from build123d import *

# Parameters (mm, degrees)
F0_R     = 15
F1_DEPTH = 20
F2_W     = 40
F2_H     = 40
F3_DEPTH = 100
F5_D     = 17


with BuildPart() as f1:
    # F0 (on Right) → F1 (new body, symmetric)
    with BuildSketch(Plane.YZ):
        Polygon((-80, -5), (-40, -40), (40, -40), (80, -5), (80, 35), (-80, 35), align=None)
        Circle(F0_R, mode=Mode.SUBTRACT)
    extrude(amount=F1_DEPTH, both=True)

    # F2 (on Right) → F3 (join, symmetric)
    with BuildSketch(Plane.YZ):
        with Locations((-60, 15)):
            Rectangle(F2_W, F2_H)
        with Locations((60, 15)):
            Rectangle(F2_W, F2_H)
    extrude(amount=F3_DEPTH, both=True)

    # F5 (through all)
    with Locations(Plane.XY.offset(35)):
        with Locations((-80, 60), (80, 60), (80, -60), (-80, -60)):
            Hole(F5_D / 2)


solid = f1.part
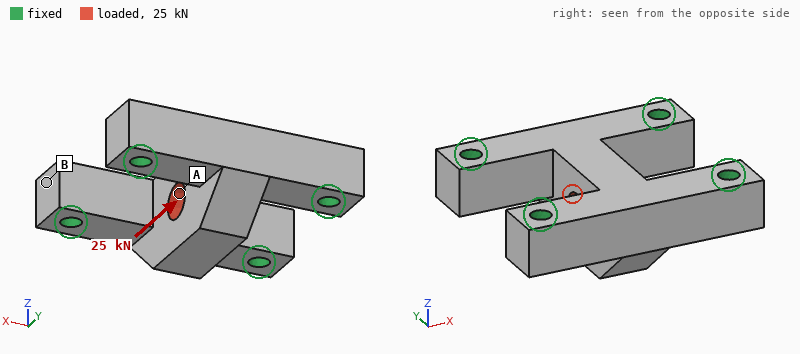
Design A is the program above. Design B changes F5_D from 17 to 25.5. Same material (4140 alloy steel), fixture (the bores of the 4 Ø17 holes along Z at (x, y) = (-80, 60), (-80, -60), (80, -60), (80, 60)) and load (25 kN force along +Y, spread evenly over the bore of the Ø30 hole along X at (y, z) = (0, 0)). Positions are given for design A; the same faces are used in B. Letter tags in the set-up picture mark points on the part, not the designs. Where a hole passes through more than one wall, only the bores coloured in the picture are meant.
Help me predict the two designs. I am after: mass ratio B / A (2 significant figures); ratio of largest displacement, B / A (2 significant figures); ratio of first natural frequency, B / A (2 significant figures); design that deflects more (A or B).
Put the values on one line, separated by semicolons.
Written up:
0.95; 0.83; 1.1; A
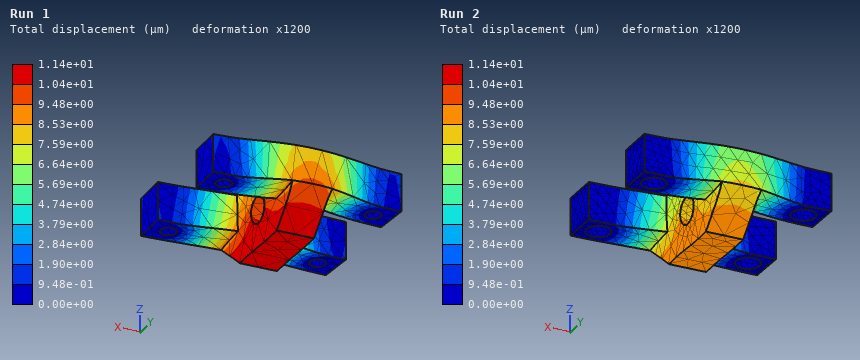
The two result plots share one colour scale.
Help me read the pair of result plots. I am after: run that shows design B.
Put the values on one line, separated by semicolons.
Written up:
Run 2
